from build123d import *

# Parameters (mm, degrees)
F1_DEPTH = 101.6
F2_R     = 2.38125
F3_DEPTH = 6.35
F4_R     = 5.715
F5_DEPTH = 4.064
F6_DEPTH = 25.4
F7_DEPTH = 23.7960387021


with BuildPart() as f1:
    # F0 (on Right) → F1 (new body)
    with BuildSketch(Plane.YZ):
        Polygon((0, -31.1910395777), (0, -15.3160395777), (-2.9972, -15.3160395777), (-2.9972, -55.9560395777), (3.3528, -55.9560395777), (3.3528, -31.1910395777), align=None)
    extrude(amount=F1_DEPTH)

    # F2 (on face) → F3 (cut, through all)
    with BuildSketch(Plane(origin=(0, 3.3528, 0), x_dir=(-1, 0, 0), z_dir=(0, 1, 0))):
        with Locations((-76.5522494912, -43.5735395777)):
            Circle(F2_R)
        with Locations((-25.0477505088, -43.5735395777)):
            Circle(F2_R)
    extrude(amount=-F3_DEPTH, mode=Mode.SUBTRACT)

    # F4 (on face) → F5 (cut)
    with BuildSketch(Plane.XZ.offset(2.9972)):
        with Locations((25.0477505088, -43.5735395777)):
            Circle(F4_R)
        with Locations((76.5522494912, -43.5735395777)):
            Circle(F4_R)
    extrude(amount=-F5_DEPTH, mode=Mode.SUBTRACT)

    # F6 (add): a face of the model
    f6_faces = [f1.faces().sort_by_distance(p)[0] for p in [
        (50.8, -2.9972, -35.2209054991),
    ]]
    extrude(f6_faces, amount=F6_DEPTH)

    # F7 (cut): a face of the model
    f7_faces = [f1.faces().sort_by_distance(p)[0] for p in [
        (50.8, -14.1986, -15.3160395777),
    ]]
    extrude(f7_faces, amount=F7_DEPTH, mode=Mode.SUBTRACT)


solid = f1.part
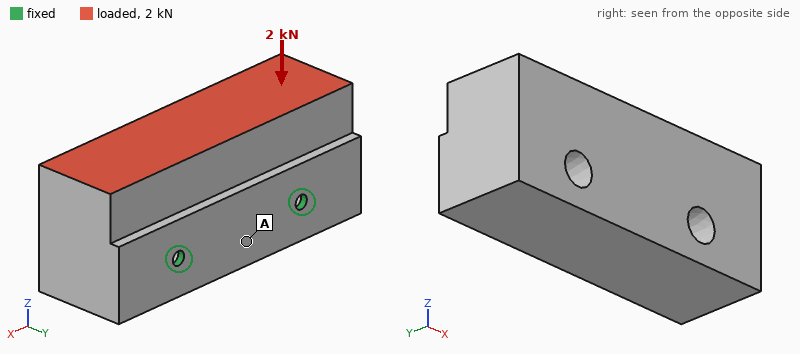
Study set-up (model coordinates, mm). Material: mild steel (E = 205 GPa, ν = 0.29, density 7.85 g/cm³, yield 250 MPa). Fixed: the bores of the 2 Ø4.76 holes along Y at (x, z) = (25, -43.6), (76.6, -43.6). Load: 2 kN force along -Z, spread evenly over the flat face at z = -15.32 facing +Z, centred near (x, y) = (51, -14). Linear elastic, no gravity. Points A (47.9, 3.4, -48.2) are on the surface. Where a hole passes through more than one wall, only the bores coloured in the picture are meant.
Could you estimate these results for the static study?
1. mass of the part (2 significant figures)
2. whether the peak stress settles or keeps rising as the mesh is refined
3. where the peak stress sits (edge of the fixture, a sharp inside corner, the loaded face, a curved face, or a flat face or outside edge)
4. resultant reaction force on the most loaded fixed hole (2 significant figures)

940 g
keeps rising
edge of the fixture
1.0 kN
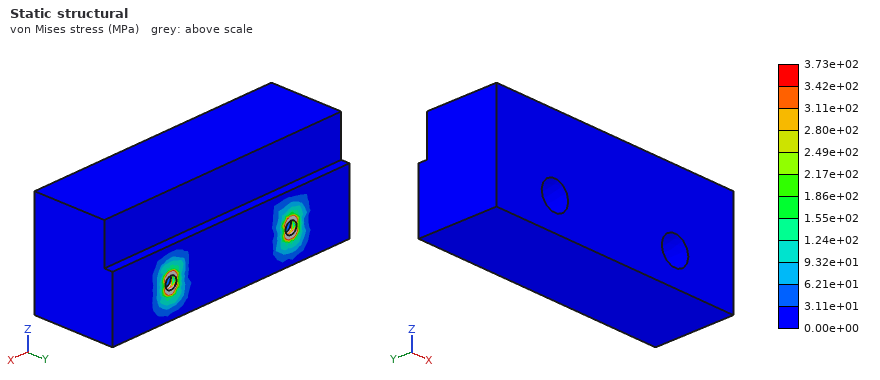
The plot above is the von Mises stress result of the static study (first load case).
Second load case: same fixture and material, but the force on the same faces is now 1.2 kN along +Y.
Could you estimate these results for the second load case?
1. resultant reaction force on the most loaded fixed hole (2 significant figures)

600 N
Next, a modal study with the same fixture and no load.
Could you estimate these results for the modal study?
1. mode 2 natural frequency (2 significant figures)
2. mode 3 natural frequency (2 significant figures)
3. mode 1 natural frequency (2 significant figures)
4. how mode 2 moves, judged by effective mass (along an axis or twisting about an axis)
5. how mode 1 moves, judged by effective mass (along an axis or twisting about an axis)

3500 Hz
4900 Hz
730 Hz
along X
along Z
